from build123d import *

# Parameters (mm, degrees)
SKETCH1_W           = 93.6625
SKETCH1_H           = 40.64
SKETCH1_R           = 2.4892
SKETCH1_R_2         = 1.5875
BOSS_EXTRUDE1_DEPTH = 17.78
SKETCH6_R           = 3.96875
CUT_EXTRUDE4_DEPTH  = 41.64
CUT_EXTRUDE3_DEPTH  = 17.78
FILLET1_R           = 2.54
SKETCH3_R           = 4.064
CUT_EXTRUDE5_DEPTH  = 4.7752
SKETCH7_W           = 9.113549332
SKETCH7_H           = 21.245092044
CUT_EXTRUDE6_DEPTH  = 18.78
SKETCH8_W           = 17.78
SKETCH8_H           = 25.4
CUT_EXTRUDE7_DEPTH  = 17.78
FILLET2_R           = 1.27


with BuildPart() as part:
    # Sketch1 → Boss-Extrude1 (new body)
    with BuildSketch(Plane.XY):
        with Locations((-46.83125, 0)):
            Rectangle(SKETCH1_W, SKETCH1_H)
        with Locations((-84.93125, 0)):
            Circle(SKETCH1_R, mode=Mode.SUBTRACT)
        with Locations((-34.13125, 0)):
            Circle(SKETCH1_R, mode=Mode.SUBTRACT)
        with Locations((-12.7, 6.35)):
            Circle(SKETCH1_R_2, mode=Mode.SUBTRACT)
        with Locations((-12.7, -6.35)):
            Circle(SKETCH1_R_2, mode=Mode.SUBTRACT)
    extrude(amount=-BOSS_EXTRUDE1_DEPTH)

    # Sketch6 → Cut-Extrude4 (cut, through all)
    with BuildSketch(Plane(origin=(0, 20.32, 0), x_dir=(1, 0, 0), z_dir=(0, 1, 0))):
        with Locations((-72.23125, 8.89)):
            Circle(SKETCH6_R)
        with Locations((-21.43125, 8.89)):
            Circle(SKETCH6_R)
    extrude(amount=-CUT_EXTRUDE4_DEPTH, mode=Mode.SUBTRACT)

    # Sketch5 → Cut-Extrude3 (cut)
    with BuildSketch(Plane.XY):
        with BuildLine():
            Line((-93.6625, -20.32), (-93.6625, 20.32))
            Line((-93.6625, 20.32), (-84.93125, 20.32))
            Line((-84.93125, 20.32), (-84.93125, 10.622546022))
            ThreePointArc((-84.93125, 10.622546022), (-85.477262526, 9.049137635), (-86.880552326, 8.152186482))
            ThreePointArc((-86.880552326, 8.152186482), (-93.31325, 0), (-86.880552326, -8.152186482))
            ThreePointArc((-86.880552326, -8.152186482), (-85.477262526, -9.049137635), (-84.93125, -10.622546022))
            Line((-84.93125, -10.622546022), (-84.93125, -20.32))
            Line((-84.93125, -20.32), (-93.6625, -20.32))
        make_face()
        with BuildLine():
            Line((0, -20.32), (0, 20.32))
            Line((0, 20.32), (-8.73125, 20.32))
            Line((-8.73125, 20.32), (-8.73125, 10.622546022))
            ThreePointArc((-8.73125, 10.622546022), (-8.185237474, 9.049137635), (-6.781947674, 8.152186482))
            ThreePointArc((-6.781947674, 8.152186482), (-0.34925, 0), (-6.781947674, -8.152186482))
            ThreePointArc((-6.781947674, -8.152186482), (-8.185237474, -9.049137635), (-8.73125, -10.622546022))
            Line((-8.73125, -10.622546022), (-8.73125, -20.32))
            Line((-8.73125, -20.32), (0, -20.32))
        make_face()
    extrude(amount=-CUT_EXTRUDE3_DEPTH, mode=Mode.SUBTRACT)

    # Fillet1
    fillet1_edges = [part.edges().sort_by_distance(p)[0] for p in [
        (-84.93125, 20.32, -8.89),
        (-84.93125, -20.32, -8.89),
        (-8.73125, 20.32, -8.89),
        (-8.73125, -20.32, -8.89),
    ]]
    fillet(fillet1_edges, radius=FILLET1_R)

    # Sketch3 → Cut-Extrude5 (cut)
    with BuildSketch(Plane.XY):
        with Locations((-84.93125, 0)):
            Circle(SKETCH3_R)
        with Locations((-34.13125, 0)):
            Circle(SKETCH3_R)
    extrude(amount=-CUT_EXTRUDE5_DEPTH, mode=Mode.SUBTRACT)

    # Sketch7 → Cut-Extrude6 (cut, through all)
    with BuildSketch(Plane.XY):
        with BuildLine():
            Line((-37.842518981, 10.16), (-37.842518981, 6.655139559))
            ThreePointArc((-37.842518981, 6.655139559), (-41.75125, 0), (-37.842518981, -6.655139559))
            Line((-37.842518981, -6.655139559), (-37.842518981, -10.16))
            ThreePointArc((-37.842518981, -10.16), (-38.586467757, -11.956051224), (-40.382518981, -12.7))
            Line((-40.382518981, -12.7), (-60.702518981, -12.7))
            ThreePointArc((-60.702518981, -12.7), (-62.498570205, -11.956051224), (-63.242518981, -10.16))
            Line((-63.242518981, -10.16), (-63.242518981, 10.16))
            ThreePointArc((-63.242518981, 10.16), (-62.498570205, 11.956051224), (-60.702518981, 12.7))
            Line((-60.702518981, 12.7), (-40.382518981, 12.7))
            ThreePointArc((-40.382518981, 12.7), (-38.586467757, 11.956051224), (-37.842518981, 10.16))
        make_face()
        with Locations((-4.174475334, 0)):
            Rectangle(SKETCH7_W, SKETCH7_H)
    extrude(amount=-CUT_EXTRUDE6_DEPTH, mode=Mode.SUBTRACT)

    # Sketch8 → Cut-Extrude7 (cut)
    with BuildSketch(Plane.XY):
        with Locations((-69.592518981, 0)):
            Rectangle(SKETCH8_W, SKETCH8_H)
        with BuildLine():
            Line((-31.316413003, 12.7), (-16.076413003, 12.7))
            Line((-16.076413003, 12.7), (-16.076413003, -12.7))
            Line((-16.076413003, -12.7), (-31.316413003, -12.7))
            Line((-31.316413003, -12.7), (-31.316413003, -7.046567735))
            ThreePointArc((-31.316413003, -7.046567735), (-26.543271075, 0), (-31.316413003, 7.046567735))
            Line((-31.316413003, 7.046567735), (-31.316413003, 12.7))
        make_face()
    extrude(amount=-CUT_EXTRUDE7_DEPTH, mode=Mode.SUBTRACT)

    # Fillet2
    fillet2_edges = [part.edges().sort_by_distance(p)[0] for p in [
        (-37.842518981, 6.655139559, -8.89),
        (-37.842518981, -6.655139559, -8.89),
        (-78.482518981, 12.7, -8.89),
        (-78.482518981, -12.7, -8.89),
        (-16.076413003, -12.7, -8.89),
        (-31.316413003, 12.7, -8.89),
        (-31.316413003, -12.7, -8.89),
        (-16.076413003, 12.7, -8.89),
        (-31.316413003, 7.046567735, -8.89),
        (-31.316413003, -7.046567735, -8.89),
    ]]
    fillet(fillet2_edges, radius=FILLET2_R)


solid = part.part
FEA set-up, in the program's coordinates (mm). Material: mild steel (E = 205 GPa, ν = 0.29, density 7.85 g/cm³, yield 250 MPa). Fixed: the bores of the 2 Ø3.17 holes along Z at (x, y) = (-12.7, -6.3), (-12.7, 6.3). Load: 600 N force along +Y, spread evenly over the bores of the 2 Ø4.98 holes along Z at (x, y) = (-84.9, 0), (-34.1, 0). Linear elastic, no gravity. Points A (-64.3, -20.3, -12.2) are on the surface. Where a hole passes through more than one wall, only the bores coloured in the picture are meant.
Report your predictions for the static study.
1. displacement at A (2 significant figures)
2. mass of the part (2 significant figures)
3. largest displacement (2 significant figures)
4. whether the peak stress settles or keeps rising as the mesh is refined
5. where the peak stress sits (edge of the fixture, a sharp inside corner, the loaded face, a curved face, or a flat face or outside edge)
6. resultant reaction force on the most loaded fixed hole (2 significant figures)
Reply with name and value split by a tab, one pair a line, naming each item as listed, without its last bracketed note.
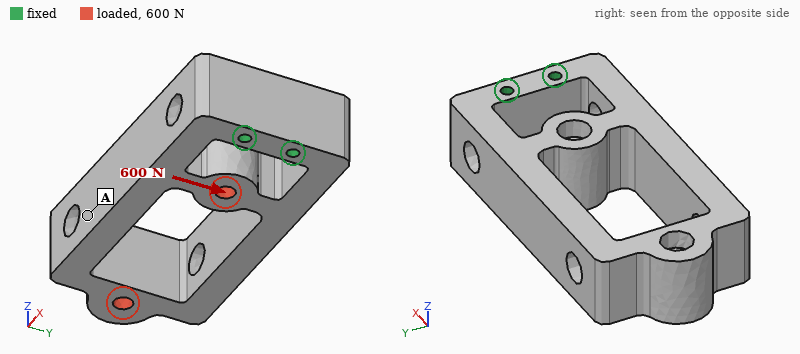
displacement at A	40 µm
mass of the part	240 g
largest displacement	55 µm
whether the peak stress settles or keeps rising as the mesh is refined	keeps rising
where the peak stress sits	edge of the fixture
resultant reaction force on the most loaded fixed hole	1.1 kN
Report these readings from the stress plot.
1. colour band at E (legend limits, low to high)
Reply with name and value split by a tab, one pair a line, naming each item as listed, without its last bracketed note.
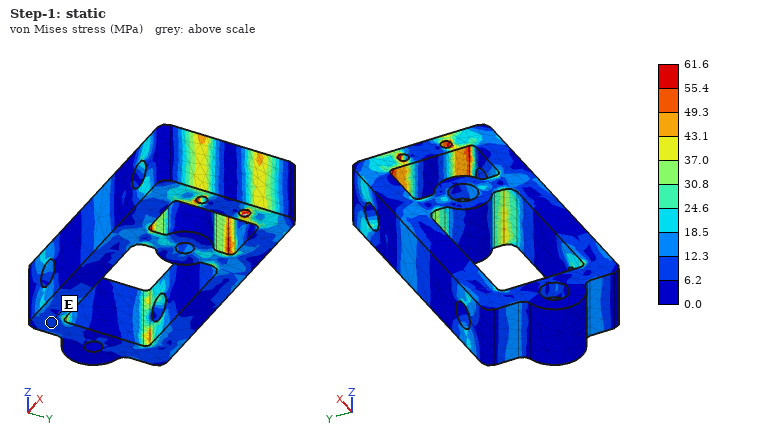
colour band at E	6.2 to 12.3 MPa
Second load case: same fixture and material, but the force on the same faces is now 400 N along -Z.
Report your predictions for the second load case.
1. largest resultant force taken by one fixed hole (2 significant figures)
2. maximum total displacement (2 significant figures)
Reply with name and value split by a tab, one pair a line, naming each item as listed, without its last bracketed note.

largest resultant force taken by one fixed hole	200 N
maximum total displacement	52 µm
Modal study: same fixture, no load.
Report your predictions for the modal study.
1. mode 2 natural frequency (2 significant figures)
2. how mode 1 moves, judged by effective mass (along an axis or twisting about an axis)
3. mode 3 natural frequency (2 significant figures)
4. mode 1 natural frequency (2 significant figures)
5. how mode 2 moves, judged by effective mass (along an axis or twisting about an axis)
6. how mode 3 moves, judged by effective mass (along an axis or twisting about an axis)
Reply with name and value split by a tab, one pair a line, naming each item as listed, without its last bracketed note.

mode 2 natural frequency	1500 Hz
how mode 1 moves, judged by effective mass	along Z
mode 3 natural frequency	3800 Hz
mode 1 natural frequency	1300 Hz
how mode 2 moves, judged by effective mass	along Y
how mode 3 moves, judged by effective mass	twisting about X
